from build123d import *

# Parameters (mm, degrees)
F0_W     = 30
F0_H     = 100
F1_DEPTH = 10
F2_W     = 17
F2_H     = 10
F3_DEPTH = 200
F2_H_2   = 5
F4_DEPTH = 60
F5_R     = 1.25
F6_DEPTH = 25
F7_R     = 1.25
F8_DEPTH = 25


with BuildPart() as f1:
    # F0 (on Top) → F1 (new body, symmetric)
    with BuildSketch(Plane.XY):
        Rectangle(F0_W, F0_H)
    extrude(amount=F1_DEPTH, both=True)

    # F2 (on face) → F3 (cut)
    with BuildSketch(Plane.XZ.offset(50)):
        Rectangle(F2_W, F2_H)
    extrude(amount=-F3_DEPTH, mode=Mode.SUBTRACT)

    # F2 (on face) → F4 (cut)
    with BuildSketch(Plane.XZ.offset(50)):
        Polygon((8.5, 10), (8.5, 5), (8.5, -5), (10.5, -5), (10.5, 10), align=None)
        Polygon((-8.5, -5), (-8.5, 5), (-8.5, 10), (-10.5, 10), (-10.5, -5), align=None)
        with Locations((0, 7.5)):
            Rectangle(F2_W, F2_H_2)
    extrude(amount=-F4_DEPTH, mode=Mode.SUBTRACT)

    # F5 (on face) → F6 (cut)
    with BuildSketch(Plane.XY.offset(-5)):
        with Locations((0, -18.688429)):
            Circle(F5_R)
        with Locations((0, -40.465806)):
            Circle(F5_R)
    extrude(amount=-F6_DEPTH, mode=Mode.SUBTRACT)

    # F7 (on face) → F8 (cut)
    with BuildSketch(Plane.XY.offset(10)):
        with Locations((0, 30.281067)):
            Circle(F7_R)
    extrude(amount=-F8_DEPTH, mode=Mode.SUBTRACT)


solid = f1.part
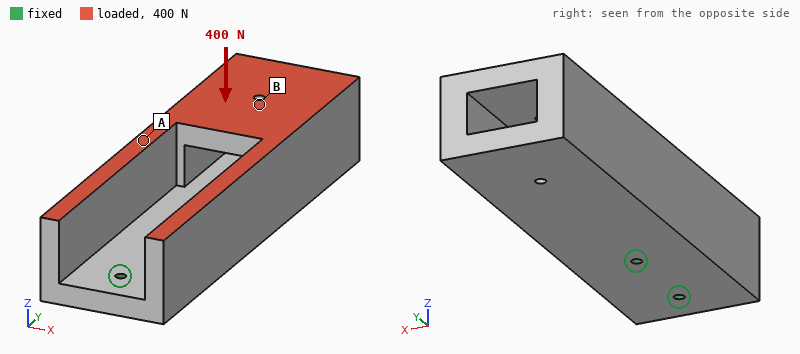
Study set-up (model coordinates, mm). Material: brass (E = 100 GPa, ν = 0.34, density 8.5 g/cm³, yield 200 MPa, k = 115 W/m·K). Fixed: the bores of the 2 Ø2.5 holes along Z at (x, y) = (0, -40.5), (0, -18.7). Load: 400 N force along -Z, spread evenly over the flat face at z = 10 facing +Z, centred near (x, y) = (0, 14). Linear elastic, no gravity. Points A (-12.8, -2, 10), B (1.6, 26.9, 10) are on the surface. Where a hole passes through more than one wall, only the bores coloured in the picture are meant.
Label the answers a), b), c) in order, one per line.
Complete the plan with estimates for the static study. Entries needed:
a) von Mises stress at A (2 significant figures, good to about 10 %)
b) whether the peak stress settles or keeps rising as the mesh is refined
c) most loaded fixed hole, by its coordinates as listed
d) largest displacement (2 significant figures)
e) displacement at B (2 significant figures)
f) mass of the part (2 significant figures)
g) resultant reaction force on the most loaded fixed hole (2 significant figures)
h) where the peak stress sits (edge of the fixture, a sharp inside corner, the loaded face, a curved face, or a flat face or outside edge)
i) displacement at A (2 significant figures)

a) 13 MPa
b) keeps rising
c) (0, -18.7)
d) 68 µm
e) 47 µm
f) 290 g
g) 880 N
h) edge of the fixture
i) 22 µm
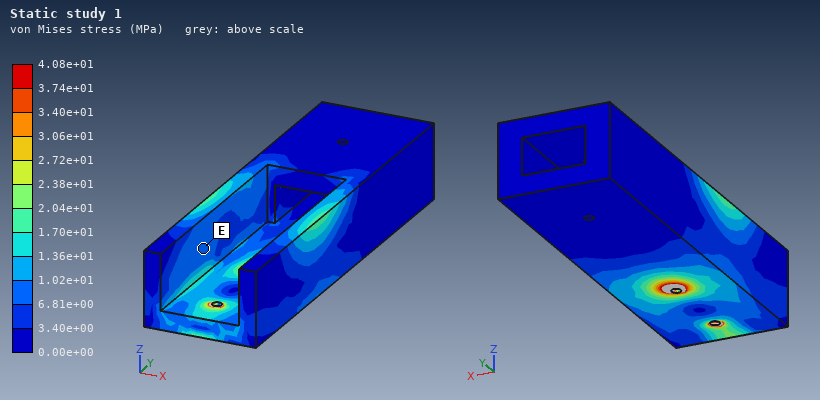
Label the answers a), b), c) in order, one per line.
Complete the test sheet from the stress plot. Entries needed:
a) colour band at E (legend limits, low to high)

a) 6.81e+00 to 1.02e+01 MPa
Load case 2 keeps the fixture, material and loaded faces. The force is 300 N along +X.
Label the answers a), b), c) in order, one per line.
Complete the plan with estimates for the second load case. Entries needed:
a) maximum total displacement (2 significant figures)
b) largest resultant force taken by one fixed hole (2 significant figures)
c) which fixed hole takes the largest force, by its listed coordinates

a) 41 µm
b) 720 N
c) (0, -18.7)
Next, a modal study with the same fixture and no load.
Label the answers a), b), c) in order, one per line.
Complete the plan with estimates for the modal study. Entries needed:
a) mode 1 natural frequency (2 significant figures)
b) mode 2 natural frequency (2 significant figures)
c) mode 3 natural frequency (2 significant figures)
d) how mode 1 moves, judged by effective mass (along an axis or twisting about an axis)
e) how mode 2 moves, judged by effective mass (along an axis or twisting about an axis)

a) 970 Hz
b) 1400 Hz
c) 1900 Hz
d) along Z
e) along X
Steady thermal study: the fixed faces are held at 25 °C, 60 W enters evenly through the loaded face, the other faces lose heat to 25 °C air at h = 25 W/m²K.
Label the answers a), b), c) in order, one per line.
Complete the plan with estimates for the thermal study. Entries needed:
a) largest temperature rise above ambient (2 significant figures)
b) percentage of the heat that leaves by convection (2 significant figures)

a) 71 K
b) 22 %
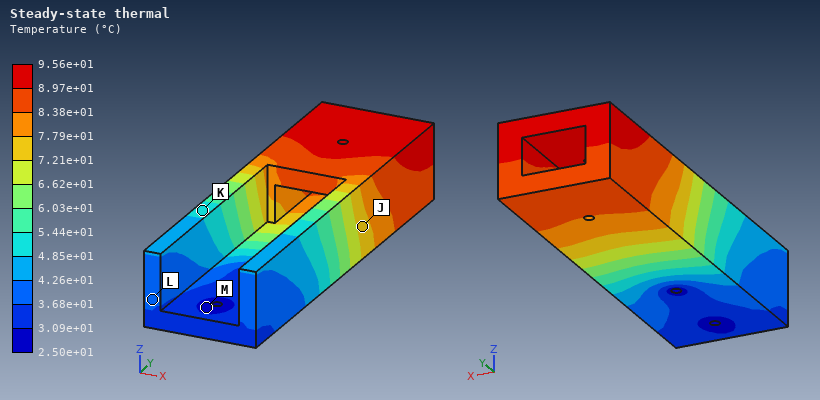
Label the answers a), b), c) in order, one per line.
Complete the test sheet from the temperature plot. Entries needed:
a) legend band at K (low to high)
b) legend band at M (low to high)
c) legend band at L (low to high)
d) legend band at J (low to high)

a) 4.85e+01 to 5.44e+01 °C
b) 2.50e+01 to 3.09e+01 °C
c) 3.68e+01 to 4.26e+01 °C
d) 7.21e+01 to 7.79e+01 °C
